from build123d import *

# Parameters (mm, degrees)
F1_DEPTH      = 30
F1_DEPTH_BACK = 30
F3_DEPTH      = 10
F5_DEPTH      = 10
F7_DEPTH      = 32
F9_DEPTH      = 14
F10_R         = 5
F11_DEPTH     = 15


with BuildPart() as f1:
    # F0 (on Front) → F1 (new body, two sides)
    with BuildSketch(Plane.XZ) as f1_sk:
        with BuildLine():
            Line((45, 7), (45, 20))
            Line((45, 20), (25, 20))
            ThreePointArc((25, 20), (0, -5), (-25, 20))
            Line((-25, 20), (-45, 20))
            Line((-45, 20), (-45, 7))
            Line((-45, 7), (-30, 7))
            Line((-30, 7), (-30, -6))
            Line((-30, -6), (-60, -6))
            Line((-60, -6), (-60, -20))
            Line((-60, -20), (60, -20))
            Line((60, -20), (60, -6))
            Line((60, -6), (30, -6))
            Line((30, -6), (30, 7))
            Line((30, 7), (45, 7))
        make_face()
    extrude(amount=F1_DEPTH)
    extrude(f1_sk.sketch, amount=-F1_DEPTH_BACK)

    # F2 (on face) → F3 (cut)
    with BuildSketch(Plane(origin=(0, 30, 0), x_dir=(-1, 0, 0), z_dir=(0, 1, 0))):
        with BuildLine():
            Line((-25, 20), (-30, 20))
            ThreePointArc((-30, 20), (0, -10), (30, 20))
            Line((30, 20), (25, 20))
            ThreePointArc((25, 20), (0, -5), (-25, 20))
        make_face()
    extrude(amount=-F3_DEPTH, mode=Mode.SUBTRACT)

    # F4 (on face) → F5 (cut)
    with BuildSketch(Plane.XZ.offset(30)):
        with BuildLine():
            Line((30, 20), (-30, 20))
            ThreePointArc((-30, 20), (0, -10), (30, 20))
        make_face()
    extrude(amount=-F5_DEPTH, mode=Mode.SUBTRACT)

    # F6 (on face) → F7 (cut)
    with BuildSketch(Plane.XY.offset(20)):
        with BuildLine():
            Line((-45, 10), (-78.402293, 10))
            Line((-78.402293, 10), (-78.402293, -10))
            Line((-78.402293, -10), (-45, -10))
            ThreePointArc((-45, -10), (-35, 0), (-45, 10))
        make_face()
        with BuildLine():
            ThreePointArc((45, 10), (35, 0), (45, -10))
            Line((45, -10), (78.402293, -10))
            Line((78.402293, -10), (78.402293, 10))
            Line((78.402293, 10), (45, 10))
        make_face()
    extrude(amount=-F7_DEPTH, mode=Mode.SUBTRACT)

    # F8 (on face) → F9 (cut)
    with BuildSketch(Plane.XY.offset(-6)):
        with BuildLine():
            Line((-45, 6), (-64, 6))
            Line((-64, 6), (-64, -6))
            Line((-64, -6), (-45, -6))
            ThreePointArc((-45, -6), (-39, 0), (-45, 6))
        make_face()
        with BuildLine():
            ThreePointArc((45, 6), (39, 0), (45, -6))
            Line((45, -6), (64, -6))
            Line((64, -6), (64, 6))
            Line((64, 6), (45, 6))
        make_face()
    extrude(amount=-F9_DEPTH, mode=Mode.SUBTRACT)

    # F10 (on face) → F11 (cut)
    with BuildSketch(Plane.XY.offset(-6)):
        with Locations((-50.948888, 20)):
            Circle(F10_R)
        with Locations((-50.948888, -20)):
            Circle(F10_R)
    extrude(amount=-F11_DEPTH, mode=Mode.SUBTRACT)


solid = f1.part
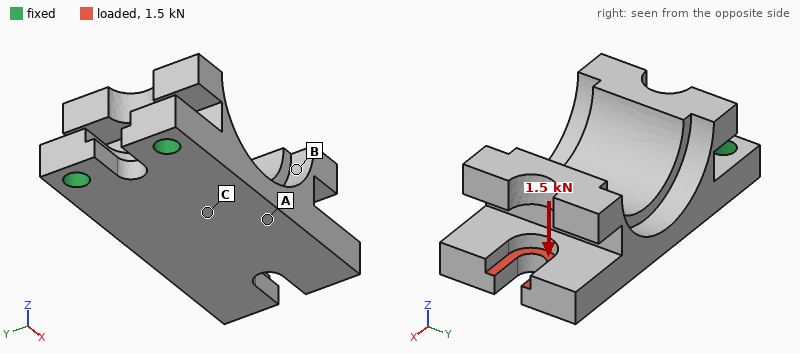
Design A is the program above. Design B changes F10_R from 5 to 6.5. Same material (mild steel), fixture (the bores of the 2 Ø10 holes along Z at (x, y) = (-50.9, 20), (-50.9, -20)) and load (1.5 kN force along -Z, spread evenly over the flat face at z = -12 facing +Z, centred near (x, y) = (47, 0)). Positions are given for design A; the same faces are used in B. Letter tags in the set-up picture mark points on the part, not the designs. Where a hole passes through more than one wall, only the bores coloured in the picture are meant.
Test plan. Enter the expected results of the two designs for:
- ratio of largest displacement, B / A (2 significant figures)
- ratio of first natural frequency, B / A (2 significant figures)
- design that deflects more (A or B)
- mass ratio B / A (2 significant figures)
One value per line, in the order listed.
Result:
0.92
1.1
A
0.99
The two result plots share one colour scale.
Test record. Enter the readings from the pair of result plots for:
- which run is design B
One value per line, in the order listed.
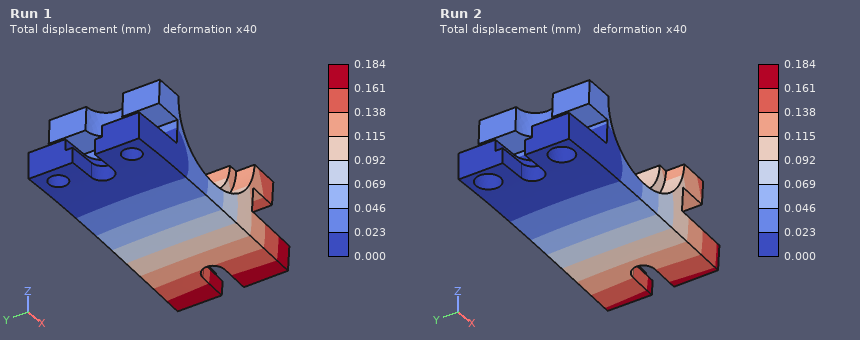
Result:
Run 2
